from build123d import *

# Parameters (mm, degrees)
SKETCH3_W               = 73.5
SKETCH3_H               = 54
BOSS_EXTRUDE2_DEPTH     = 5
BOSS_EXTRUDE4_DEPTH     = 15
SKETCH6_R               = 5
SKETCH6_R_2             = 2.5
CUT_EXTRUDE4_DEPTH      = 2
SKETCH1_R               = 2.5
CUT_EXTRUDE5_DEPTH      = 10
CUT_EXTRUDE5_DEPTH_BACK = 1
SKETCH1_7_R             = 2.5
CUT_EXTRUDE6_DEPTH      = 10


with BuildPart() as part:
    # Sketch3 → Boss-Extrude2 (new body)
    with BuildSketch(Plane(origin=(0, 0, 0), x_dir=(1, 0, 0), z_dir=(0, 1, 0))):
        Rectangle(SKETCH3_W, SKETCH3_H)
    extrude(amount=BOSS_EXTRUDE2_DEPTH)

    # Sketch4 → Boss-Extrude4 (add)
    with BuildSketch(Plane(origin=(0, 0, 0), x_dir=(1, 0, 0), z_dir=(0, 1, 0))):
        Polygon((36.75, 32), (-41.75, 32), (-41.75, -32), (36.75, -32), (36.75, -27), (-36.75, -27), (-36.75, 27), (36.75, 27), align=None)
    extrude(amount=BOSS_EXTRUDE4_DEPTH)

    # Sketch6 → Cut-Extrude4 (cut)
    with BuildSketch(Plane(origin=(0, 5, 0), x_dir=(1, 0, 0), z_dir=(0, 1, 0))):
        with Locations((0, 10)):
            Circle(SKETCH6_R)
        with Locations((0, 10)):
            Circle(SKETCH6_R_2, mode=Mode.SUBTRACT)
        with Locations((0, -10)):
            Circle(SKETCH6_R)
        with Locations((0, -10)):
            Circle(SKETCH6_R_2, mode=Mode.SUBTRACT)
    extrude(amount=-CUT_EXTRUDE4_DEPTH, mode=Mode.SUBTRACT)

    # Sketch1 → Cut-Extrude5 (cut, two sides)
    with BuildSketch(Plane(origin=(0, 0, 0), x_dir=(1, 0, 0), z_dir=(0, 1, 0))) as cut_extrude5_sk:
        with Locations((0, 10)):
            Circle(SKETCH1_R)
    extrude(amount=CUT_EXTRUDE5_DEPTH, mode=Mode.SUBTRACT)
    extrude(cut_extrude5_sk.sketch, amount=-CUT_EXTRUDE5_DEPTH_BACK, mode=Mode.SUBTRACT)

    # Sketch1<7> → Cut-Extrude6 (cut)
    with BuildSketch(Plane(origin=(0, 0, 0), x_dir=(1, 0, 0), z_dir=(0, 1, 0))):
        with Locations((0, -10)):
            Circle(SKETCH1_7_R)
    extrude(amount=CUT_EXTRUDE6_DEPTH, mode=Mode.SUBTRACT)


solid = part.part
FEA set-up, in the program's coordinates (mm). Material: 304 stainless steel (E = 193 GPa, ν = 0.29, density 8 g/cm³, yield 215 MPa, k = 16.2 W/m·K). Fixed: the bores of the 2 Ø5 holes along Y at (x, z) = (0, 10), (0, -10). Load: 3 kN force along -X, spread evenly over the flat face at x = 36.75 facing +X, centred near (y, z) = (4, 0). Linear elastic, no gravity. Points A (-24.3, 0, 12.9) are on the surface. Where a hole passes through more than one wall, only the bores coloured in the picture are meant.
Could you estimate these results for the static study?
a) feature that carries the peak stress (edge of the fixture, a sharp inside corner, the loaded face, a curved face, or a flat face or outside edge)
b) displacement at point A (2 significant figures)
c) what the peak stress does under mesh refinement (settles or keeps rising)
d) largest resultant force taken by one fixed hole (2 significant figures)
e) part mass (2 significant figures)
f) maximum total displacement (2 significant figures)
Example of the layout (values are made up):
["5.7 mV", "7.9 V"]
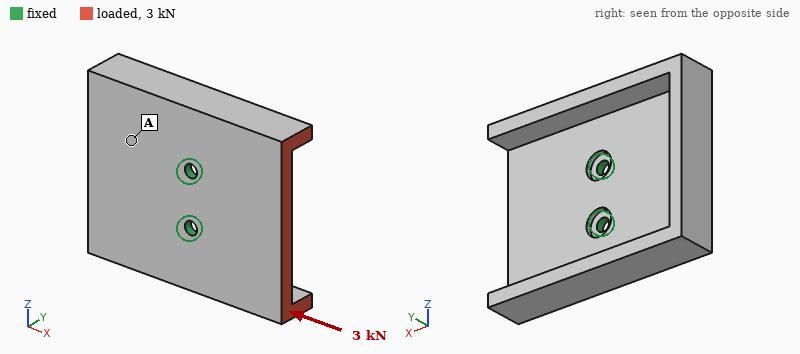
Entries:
["edge of the fixture", "19 µm", "keeps rising", "1.5 kN", "280 g", "37 µm"]
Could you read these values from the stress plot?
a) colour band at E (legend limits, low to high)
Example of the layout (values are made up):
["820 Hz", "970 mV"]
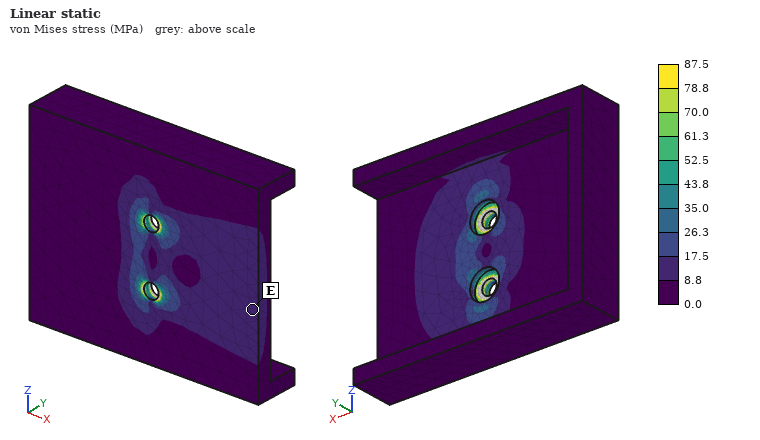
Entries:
["8.8 to 17.5 MPa"]
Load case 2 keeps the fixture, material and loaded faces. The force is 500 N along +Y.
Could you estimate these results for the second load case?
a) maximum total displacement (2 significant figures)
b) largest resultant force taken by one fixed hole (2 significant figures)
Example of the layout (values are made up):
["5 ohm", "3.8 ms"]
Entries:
["85 µm", "350 N"]
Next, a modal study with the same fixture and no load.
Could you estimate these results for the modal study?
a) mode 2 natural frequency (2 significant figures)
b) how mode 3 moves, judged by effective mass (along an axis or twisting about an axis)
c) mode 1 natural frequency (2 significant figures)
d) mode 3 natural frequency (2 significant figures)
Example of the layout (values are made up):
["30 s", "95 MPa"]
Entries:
["2400 Hz", "twisting about X", "1200 Hz", "2900 Hz"]
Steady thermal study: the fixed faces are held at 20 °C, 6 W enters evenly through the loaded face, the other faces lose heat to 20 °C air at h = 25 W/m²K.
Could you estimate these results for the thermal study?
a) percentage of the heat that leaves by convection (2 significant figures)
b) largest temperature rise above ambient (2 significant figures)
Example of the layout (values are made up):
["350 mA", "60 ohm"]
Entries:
["55 %", "29 K"]
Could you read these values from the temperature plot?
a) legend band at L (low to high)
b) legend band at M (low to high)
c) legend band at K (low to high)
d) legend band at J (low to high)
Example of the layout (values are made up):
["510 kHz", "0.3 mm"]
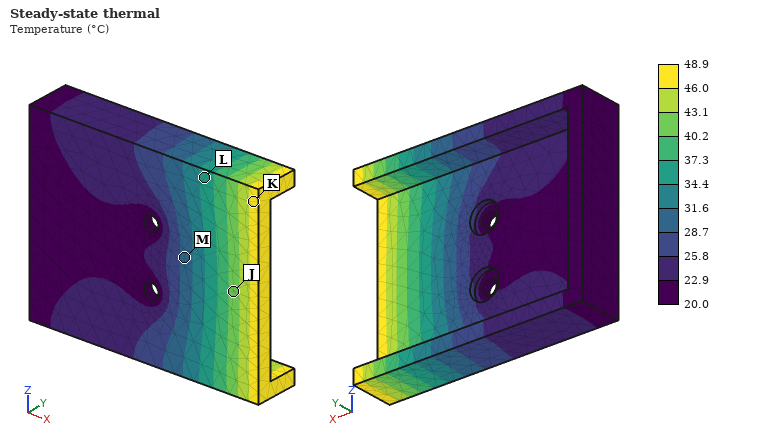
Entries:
["34.4 to 37.3 °C", "28.7 to 31.6 °C", "46.0 to 48.9 °C", "40.2 to 43.1 °C"]
